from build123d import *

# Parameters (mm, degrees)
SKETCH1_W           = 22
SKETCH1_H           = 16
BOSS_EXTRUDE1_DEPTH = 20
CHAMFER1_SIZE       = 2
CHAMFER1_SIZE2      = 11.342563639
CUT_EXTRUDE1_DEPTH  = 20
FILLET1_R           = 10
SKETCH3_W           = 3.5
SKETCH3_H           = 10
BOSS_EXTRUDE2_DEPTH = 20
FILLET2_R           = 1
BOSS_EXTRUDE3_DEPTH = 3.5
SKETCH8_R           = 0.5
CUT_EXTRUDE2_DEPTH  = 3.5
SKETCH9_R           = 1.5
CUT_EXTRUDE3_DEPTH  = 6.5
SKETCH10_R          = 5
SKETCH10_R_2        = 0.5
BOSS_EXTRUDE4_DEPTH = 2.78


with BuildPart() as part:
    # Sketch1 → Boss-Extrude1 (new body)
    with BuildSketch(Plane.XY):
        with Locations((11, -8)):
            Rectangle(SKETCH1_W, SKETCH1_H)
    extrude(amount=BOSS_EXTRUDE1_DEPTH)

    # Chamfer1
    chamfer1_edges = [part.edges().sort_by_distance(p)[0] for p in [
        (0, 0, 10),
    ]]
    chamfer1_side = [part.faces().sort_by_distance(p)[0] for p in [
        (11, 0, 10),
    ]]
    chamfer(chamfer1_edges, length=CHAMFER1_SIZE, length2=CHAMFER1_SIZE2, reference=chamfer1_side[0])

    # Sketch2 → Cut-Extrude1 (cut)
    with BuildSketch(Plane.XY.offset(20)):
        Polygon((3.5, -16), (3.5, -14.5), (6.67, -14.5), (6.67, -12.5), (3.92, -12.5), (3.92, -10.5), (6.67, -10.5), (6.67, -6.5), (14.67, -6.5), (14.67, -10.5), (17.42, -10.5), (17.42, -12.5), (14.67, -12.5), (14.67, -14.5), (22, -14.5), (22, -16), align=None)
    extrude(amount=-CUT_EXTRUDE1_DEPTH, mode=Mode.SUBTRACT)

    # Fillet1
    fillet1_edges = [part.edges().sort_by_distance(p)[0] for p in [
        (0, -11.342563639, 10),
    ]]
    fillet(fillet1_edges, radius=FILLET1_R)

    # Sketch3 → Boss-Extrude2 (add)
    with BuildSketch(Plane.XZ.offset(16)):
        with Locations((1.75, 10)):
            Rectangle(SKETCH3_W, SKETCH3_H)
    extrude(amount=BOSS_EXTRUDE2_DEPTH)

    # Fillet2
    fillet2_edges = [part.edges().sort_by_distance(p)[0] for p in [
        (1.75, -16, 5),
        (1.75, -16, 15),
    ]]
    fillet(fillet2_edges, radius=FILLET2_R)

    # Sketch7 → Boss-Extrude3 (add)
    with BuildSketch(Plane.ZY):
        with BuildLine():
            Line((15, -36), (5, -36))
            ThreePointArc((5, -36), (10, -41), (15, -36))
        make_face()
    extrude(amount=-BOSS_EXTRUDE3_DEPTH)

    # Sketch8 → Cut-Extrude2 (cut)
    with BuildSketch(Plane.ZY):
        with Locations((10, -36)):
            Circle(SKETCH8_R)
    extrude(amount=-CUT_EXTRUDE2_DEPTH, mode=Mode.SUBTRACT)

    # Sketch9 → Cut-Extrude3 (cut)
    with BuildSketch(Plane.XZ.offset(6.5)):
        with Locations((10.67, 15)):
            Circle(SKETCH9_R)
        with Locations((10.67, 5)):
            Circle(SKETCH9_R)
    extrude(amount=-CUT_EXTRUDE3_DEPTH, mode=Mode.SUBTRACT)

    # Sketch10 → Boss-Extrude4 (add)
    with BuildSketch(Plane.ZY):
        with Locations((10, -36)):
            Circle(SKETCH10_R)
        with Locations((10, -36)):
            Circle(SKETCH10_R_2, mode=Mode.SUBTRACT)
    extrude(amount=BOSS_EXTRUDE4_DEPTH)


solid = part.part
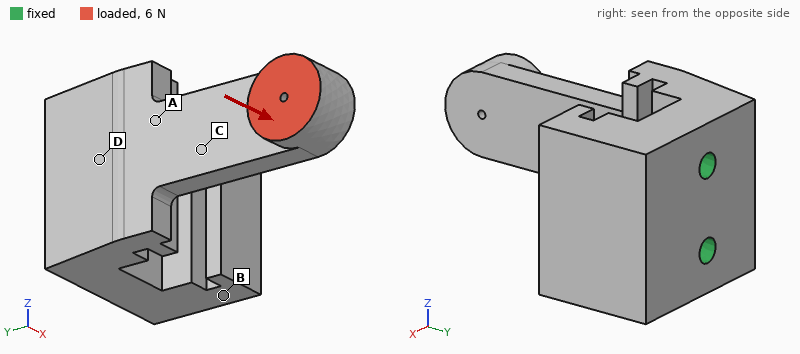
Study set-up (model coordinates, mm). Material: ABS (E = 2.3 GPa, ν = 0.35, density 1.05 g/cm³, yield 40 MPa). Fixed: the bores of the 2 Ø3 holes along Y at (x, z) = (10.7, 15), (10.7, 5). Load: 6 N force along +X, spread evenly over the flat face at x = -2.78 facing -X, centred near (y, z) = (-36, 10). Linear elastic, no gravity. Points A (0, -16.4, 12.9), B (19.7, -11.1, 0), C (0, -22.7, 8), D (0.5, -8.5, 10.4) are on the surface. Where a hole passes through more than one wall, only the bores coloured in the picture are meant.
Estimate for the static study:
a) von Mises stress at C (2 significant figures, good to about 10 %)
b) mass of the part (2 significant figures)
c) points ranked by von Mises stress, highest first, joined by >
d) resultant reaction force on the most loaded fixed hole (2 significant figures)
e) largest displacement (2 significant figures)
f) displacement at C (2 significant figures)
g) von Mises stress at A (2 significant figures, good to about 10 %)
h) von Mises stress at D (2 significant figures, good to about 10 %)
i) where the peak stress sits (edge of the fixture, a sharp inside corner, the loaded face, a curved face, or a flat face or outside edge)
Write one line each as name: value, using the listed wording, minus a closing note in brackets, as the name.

von Mises stress at C: 3.9 MPa
mass of the part: 6.0 g
points ranked by von Mises stress, highest first, joined by >: A > C > D > B
resultant reaction force on the most loaded fixed hole: 4.1 N
largest displacement: 0.53 mm
displacement at C: 0.14 mm
von Mises stress at A: 5.1 MPa
von Mises stress at D: 2.3 MPa
where the peak stress sits: a curved face
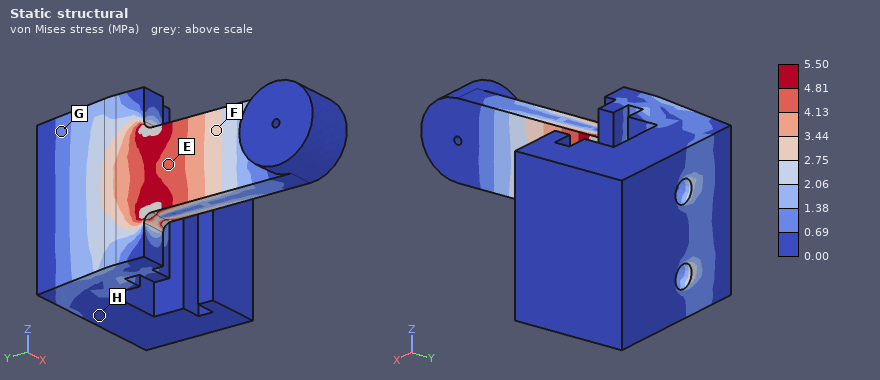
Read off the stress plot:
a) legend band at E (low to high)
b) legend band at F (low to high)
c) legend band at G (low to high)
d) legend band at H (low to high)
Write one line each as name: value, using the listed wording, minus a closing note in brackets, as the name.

legend band at E: 4.13 to 4.81 MPa
legend band at F: 2.75 to 3.44 MPa
legend band at G: 0.69 to 1.38 MPa
legend band at H: 0.00 to 0.69 MPa
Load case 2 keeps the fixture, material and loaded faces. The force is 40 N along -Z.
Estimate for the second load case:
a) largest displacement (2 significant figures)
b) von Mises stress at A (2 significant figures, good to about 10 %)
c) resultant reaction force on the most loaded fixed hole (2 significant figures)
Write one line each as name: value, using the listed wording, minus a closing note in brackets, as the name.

largest displacement: 0.61 mm
von Mises stress at A: 6.7 MPa
resultant reaction force on the most loaded fixed hole: 100 N
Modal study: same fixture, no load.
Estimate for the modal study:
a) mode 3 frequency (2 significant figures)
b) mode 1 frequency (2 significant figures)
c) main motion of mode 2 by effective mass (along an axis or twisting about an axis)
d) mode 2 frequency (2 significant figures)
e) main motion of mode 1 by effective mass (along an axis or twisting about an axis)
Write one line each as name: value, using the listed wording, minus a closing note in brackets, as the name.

mode 3 frequency: 3900 Hz
mode 1 frequency: 750 Hz
main motion of mode 2 by effective mass: along Z
mode 2 frequency: 1900 Hz
main motion of mode 1 by effective mass: along X
